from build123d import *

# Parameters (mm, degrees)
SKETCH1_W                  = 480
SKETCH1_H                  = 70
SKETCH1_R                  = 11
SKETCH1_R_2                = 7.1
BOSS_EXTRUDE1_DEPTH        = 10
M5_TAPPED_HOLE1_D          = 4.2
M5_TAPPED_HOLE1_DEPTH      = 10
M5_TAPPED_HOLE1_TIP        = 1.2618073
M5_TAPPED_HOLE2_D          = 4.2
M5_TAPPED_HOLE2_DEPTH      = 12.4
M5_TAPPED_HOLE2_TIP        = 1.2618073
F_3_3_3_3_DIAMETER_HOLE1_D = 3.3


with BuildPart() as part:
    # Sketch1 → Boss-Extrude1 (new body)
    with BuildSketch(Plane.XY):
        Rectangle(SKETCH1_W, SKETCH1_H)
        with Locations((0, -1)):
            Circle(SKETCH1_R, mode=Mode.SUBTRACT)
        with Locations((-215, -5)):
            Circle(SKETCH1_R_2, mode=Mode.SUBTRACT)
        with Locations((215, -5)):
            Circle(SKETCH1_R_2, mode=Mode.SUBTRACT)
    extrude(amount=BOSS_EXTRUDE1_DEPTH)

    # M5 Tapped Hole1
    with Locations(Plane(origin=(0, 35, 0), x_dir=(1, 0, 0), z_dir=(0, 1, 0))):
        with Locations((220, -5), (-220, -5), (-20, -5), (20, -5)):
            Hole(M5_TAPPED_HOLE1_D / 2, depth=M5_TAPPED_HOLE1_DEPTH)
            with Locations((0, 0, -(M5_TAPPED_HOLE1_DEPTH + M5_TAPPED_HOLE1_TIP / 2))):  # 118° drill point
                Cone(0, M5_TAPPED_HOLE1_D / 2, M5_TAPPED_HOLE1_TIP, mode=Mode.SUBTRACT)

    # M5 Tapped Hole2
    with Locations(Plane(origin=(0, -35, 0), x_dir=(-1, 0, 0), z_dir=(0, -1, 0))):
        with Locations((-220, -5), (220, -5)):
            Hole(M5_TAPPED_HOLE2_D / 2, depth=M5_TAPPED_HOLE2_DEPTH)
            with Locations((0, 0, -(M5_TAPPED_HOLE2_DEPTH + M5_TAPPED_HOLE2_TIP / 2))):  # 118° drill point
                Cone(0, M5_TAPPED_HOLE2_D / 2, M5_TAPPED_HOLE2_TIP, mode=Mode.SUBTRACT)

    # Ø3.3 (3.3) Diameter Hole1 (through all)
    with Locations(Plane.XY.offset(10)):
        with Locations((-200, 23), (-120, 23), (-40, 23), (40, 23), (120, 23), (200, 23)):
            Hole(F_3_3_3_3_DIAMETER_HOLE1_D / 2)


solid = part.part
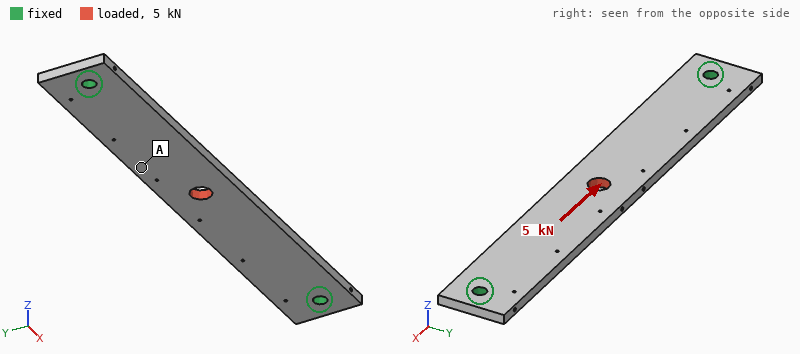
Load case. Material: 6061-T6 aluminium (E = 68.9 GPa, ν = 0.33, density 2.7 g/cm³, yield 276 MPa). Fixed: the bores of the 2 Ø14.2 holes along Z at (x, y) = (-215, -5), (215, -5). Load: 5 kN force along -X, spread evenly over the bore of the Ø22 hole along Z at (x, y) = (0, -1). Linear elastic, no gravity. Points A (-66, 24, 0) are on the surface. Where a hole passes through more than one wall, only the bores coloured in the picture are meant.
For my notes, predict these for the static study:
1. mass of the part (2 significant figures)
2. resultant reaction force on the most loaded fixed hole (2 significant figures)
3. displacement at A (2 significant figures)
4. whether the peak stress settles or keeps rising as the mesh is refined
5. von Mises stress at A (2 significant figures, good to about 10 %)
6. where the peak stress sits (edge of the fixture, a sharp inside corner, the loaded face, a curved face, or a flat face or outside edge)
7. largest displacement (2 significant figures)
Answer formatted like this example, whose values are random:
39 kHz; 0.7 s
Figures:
880 g; 2.5 kN; 8.7 µm; keeps rising; 3.2 MPa; edge of the fixture; 13 µm
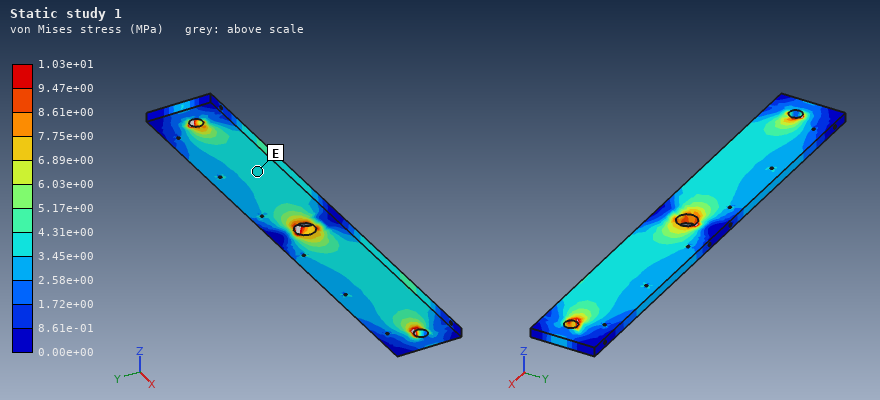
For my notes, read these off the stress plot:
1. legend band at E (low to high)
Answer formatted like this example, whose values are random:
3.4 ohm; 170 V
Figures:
3.45e+00 to 4.31e+00 MPa
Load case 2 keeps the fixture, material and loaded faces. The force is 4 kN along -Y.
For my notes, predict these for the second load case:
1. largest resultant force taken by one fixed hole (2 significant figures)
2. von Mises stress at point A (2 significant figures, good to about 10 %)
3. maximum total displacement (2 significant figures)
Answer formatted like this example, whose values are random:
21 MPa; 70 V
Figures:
2.2 kN; 15 MPa; 0.20 mm
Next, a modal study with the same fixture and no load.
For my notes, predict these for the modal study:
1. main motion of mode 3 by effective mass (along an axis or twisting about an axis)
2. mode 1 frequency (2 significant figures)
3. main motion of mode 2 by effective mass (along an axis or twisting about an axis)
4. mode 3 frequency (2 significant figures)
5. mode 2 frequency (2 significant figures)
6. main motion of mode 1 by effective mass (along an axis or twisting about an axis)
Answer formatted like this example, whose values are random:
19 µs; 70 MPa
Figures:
twisting about X; 280 Hz; twisting about Y; 1000 Hz; 780 Hz; along Z
